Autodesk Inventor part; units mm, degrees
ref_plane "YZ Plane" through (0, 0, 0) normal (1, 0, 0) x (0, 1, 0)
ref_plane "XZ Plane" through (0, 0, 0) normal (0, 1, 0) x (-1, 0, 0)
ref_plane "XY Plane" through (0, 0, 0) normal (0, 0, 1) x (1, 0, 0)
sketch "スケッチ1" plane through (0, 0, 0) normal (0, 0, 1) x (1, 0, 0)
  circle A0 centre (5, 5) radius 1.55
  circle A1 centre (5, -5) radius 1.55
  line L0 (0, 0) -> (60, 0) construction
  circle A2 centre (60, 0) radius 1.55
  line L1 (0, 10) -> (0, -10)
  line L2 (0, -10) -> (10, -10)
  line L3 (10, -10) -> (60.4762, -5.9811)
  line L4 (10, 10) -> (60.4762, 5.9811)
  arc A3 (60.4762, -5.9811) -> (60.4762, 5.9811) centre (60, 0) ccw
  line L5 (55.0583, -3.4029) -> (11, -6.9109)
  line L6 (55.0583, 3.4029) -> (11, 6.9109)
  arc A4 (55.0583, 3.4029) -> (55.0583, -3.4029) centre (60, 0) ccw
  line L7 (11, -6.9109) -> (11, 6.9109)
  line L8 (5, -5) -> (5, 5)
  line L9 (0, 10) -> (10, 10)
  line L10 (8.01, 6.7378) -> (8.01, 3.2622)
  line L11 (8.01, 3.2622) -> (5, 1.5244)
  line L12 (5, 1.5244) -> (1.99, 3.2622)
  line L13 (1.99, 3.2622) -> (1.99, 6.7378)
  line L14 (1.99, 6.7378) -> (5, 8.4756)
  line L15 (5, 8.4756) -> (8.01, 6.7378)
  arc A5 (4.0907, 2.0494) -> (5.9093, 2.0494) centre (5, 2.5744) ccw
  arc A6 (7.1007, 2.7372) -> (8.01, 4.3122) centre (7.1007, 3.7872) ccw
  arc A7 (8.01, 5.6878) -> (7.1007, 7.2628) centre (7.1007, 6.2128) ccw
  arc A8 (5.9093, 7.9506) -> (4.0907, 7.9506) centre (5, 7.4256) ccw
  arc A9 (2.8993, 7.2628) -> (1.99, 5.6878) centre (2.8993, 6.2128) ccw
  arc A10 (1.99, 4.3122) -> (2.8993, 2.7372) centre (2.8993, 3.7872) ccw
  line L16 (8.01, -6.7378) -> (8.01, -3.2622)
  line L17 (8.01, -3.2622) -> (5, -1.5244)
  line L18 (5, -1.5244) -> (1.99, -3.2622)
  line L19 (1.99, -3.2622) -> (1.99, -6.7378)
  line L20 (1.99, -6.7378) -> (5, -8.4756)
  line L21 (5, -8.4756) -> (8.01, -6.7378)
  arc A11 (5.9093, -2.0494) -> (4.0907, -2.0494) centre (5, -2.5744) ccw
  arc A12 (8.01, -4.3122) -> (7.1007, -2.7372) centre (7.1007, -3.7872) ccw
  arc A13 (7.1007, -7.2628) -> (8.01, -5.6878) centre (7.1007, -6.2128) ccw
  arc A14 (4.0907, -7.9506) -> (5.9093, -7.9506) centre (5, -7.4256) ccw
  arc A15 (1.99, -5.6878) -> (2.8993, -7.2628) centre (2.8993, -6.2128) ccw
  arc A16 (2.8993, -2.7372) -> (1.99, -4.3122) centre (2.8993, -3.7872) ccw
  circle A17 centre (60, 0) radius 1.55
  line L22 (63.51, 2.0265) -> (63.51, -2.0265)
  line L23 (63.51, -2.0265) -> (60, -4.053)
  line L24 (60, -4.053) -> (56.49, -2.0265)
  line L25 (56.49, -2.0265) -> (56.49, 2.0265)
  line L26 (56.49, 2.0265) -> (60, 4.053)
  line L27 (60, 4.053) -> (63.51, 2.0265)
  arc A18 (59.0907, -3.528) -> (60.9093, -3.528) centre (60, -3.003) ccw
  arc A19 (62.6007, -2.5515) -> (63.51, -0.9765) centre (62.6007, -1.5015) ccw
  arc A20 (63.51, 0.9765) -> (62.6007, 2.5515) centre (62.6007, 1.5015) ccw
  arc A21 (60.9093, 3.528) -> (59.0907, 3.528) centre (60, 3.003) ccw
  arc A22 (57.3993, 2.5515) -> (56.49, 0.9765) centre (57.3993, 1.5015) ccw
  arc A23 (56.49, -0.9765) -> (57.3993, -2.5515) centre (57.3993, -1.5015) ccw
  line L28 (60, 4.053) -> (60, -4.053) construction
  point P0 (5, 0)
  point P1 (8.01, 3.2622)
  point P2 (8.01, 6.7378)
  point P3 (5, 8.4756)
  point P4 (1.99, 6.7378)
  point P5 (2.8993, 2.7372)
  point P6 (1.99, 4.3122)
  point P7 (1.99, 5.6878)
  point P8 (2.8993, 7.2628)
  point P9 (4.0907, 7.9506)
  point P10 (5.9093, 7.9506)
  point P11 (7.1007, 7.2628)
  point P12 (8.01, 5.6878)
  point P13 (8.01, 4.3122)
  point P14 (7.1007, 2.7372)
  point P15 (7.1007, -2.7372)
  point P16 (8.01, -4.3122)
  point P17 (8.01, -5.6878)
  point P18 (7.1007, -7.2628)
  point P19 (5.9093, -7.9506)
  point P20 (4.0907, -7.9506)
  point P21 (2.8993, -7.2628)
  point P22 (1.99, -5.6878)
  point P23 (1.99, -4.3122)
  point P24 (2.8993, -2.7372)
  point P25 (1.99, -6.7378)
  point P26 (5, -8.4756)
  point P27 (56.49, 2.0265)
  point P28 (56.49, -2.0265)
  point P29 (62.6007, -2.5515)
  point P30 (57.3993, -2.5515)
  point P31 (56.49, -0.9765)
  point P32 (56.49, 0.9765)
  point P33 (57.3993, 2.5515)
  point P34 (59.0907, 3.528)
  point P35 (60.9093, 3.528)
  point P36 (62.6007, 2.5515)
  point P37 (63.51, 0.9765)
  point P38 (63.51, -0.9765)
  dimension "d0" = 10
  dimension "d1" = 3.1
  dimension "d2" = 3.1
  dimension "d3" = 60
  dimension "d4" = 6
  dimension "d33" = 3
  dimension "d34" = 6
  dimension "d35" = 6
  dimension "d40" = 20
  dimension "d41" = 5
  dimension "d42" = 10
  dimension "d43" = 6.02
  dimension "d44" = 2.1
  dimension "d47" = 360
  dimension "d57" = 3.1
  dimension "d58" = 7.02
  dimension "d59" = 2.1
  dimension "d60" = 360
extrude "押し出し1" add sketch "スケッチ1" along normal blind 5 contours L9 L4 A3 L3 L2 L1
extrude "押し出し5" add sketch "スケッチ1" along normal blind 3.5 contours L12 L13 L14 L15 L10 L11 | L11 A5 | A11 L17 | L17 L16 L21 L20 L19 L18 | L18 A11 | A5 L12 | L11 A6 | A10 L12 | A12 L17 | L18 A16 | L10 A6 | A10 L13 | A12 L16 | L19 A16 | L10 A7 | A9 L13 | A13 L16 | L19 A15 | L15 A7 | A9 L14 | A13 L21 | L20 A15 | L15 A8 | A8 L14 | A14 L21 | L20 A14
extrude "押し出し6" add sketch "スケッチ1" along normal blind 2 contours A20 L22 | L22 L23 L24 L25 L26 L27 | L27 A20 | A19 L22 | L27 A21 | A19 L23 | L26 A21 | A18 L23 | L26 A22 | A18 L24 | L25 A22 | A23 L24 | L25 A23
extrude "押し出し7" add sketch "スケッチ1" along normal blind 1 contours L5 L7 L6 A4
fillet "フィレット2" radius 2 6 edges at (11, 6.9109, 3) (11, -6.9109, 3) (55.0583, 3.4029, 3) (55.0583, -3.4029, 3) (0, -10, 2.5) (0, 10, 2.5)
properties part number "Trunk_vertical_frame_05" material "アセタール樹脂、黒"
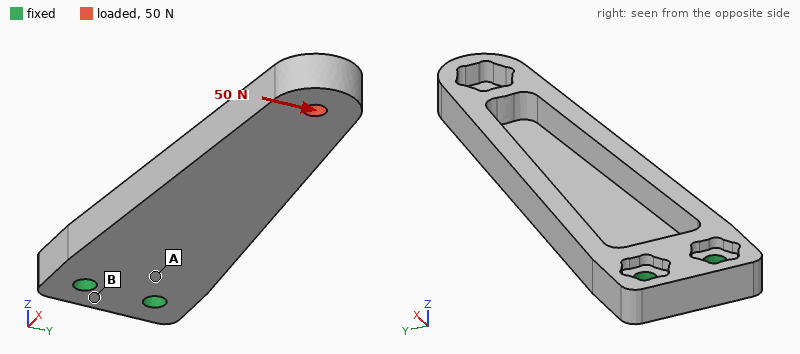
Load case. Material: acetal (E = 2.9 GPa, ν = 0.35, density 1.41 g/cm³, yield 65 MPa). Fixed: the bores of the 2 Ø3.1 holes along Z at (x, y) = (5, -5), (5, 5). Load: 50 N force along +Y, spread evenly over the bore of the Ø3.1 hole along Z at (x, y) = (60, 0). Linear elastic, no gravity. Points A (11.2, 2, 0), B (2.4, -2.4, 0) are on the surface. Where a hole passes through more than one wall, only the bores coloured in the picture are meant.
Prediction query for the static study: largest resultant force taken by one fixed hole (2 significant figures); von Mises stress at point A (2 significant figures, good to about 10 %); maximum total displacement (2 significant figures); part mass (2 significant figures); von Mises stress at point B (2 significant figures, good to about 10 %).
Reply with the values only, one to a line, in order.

220 N
6.6 MPa
0.83 mm
4.5 g
2.9 MPa
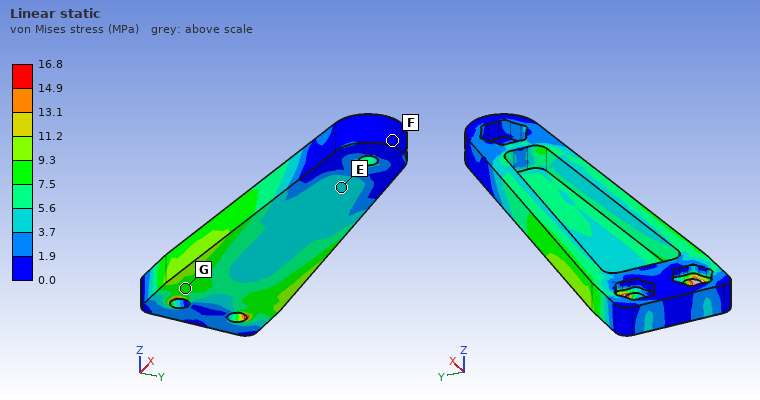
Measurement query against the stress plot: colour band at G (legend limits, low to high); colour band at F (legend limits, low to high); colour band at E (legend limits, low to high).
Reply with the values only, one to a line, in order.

7.5 to 9.3 MPa
0.0 to 1.9 MPa
3.7 to 5.6 MPa
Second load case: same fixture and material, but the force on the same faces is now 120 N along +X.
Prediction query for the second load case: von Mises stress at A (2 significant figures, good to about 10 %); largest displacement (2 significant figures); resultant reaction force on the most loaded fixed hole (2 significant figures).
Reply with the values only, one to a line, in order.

4.3 MPa
0.72 mm
60 N
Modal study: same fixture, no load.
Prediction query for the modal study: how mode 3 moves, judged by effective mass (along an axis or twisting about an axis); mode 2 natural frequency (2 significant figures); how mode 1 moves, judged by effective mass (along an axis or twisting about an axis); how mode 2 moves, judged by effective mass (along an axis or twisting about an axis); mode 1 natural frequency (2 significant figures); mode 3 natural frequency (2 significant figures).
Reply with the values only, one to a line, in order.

along Y
1000 Hz
along Z
along Y
340 Hz
1500 Hz
